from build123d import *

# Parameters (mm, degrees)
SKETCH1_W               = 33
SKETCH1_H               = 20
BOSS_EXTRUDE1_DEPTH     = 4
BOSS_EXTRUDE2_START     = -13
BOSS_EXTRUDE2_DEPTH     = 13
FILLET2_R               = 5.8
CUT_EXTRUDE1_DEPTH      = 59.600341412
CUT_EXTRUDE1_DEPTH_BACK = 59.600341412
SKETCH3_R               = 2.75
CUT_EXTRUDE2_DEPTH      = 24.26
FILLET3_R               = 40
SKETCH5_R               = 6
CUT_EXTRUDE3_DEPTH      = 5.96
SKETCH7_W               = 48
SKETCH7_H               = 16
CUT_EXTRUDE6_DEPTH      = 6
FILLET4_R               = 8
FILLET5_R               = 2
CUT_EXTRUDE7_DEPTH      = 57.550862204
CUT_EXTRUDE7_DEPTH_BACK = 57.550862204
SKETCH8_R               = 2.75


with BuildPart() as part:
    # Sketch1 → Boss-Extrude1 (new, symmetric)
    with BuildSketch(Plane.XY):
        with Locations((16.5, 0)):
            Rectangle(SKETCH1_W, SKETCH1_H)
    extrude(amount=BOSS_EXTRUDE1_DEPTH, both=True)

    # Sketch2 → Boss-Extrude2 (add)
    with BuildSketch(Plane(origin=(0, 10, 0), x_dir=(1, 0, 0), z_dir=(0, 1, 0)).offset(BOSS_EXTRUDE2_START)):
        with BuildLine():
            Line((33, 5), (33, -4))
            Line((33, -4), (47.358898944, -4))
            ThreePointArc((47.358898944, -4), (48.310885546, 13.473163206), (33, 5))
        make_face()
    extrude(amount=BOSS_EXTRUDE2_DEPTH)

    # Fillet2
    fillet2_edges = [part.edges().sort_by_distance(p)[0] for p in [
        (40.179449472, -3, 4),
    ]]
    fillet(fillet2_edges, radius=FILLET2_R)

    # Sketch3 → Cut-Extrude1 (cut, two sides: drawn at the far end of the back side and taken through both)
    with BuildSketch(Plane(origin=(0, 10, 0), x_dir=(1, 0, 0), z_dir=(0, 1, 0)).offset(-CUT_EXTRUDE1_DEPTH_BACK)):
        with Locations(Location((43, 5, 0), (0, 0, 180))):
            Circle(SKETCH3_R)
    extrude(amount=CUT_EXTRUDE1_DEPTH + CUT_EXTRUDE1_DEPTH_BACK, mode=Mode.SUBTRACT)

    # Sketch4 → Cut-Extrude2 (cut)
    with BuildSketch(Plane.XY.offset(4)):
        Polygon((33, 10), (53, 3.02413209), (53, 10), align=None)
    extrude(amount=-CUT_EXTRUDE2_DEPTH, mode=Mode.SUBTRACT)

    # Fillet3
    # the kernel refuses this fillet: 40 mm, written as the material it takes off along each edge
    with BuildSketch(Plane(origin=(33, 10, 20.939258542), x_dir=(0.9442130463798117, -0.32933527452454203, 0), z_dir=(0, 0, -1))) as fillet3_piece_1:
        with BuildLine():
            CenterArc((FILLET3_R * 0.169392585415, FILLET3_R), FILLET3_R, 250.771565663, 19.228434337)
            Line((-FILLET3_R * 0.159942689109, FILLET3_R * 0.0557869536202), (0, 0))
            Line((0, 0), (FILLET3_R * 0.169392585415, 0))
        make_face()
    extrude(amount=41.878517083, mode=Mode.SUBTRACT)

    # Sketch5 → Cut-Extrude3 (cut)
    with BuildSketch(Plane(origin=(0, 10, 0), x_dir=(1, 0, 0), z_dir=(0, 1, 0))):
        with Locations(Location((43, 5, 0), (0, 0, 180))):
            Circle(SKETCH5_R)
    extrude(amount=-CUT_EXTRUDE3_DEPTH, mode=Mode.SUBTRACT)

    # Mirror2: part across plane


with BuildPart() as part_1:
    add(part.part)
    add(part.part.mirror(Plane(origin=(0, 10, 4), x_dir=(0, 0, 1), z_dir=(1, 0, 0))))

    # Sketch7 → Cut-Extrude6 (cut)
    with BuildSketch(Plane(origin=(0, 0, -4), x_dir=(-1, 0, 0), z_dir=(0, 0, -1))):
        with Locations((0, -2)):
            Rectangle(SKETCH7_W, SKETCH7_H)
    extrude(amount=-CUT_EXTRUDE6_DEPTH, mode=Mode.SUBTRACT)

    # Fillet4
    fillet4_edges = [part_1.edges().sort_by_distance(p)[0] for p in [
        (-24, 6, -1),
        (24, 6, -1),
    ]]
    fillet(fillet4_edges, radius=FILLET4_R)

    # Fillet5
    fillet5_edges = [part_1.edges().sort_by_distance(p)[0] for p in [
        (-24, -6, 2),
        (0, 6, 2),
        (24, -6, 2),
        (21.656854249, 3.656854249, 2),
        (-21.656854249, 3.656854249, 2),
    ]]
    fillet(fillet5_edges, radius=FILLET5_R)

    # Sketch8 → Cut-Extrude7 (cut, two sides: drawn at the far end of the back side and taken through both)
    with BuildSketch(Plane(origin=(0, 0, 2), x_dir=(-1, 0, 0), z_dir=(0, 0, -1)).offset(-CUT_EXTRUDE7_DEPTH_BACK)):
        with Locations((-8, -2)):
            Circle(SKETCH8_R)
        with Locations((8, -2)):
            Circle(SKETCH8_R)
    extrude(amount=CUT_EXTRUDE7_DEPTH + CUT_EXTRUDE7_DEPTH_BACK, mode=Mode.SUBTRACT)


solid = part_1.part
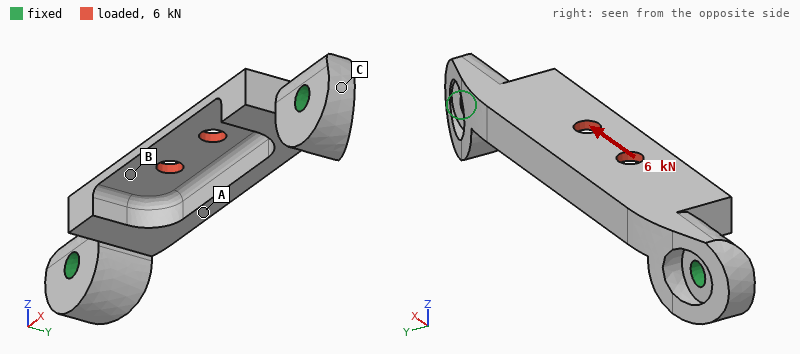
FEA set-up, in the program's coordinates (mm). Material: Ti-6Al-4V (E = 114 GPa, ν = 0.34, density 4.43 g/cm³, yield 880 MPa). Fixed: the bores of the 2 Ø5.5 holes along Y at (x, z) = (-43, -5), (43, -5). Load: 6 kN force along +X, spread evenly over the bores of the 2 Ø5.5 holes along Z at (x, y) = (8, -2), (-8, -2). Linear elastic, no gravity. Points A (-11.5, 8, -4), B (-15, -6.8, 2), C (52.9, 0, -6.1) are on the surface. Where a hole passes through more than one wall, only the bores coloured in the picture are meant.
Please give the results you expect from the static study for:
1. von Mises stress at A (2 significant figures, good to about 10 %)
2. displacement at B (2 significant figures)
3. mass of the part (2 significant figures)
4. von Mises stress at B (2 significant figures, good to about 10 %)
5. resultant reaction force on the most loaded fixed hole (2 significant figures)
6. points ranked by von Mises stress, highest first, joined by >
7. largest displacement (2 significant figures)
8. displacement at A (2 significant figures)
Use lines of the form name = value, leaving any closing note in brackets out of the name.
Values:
von Mises stress at A = 44 MPa
displacement at B = 35 µm
mass of the part = 49 g
von Mises stress at B = 110 MPa
resultant reaction force on the most loaded fixed hole = 3.0 kN
points ranked by von Mises stress, highest first, joined by > = B > A > C
largest displacement = 41 µm
displacement at A = 17 µm
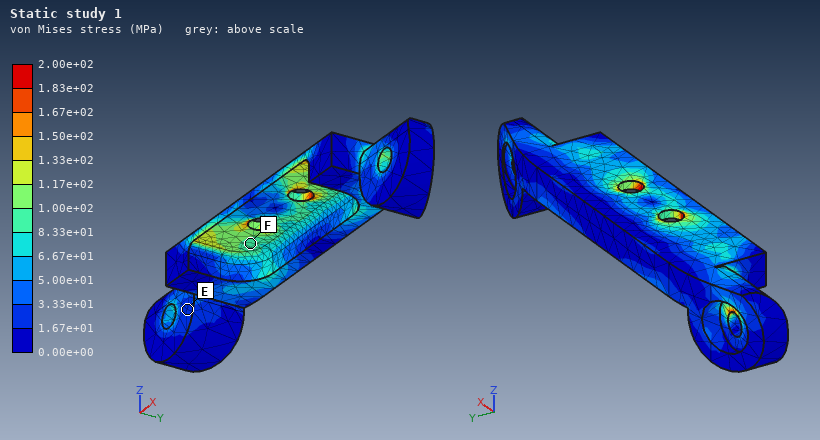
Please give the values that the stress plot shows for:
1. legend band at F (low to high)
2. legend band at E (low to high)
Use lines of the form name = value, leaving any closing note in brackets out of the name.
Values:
legend band at F = 8.33e+01 to 1.00e+02 MPa
legend band at E = 1.67e+01 to 3.33e+01 MPa
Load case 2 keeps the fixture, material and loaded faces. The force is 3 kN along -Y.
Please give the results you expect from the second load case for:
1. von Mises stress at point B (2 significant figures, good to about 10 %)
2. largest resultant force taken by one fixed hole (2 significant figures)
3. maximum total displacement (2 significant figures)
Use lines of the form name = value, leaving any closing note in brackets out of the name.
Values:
von Mises stress at point B = 85 MPa
largest resultant force taken by one fixed hole = 1.8 kN
maximum total displacement = 0.11 mm
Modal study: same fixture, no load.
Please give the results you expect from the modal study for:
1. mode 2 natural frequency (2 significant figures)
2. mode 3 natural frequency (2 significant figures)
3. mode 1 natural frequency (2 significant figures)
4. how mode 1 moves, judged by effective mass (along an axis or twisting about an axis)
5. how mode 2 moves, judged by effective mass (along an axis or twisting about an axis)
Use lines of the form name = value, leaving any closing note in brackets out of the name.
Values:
mode 2 natural frequency = 8100 Hz
mode 3 natural frequency = 9400 Hz
mode 1 natural frequency = 6100 Hz
how mode 1 moves, judged by effective mass = along Z
how mode 2 moves, judged by effective mass = along Y
